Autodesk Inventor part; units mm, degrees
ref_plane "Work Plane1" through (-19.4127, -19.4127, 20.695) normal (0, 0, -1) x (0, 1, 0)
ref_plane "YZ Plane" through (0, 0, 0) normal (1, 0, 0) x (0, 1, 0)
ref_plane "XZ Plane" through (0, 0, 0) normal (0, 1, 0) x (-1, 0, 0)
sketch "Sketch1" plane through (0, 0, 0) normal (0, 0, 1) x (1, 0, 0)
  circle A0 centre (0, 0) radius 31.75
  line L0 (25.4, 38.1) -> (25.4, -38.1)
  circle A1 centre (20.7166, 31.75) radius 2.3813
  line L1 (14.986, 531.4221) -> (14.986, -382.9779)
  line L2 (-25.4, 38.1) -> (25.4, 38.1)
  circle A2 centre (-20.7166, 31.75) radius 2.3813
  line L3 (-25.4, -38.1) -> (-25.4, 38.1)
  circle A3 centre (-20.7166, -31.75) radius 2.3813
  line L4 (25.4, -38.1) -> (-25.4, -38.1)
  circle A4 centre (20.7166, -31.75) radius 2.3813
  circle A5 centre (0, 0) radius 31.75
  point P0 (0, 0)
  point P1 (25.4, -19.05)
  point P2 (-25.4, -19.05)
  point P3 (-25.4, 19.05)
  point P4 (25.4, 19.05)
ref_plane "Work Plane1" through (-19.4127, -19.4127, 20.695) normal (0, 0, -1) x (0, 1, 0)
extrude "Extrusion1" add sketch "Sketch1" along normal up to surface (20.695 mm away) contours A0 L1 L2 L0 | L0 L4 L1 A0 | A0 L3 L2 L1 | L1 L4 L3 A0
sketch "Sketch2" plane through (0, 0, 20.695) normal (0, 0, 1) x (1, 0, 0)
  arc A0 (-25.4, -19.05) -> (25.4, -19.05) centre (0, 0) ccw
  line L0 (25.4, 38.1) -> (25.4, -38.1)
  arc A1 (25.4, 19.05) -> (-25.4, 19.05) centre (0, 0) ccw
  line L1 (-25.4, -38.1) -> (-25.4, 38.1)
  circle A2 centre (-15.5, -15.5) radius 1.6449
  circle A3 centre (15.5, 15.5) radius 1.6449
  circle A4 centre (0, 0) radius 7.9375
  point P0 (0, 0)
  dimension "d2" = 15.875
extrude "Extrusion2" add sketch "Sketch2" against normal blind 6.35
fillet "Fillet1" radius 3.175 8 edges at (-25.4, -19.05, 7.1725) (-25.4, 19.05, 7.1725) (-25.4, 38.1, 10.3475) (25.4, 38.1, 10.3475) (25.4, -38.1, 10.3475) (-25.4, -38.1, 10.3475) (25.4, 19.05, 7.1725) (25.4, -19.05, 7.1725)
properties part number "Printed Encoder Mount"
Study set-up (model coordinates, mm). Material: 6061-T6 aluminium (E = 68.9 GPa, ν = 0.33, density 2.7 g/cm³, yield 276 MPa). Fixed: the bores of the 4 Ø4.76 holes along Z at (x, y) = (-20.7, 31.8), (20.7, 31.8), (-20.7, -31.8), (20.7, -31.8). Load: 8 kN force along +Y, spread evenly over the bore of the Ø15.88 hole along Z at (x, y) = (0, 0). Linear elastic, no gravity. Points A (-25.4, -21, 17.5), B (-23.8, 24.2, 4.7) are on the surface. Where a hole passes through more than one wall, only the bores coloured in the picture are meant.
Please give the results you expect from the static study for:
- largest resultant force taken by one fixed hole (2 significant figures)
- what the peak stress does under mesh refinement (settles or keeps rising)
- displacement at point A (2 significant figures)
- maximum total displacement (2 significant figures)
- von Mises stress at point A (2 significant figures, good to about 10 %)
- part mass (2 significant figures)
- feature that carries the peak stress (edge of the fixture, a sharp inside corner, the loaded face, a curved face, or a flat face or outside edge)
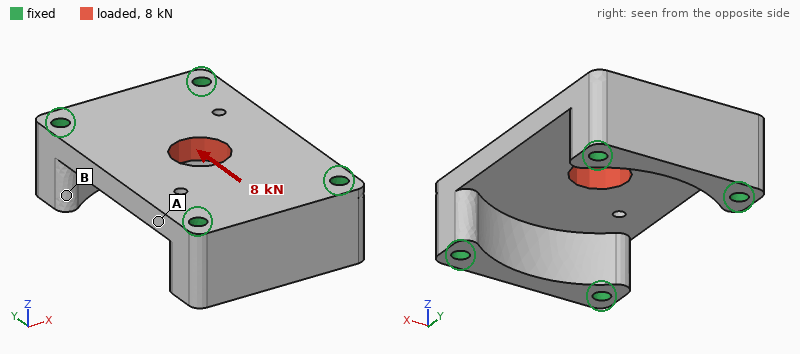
2.1 kN
keeps rising
2.6 µm
10 µm
13 MPa
96 g
edge of the fixture
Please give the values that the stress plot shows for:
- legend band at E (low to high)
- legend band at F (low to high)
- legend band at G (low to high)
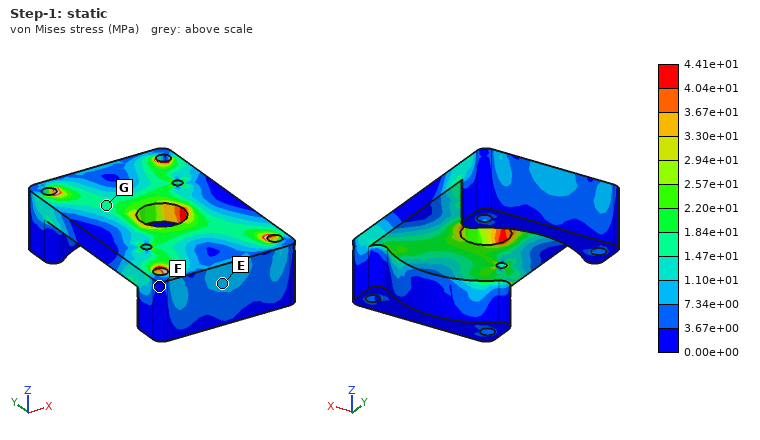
7.34e+00 to 1.10e+01 MPa
0.00e+00 to 3.67e+00 MPa
1.47e+01 to 1.84e+01 MPa
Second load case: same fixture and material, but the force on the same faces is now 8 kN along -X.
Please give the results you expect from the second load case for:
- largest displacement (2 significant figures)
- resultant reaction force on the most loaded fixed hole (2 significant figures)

19 µm
2.5 kN
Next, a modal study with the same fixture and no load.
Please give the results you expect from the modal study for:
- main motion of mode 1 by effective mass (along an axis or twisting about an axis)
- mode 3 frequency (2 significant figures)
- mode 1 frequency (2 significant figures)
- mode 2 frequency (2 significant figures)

along Z
18 kHz
8600 Hz
12 kHz
